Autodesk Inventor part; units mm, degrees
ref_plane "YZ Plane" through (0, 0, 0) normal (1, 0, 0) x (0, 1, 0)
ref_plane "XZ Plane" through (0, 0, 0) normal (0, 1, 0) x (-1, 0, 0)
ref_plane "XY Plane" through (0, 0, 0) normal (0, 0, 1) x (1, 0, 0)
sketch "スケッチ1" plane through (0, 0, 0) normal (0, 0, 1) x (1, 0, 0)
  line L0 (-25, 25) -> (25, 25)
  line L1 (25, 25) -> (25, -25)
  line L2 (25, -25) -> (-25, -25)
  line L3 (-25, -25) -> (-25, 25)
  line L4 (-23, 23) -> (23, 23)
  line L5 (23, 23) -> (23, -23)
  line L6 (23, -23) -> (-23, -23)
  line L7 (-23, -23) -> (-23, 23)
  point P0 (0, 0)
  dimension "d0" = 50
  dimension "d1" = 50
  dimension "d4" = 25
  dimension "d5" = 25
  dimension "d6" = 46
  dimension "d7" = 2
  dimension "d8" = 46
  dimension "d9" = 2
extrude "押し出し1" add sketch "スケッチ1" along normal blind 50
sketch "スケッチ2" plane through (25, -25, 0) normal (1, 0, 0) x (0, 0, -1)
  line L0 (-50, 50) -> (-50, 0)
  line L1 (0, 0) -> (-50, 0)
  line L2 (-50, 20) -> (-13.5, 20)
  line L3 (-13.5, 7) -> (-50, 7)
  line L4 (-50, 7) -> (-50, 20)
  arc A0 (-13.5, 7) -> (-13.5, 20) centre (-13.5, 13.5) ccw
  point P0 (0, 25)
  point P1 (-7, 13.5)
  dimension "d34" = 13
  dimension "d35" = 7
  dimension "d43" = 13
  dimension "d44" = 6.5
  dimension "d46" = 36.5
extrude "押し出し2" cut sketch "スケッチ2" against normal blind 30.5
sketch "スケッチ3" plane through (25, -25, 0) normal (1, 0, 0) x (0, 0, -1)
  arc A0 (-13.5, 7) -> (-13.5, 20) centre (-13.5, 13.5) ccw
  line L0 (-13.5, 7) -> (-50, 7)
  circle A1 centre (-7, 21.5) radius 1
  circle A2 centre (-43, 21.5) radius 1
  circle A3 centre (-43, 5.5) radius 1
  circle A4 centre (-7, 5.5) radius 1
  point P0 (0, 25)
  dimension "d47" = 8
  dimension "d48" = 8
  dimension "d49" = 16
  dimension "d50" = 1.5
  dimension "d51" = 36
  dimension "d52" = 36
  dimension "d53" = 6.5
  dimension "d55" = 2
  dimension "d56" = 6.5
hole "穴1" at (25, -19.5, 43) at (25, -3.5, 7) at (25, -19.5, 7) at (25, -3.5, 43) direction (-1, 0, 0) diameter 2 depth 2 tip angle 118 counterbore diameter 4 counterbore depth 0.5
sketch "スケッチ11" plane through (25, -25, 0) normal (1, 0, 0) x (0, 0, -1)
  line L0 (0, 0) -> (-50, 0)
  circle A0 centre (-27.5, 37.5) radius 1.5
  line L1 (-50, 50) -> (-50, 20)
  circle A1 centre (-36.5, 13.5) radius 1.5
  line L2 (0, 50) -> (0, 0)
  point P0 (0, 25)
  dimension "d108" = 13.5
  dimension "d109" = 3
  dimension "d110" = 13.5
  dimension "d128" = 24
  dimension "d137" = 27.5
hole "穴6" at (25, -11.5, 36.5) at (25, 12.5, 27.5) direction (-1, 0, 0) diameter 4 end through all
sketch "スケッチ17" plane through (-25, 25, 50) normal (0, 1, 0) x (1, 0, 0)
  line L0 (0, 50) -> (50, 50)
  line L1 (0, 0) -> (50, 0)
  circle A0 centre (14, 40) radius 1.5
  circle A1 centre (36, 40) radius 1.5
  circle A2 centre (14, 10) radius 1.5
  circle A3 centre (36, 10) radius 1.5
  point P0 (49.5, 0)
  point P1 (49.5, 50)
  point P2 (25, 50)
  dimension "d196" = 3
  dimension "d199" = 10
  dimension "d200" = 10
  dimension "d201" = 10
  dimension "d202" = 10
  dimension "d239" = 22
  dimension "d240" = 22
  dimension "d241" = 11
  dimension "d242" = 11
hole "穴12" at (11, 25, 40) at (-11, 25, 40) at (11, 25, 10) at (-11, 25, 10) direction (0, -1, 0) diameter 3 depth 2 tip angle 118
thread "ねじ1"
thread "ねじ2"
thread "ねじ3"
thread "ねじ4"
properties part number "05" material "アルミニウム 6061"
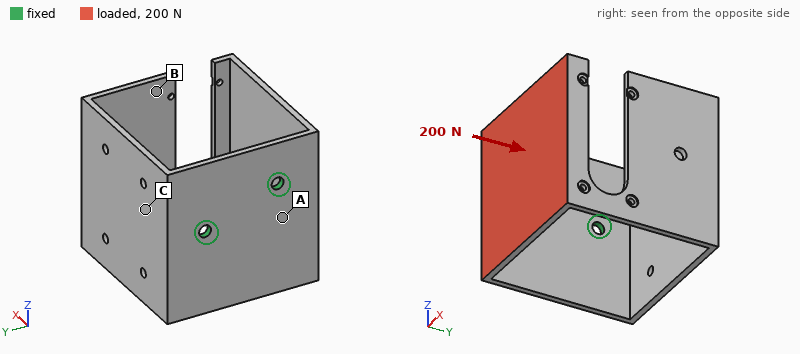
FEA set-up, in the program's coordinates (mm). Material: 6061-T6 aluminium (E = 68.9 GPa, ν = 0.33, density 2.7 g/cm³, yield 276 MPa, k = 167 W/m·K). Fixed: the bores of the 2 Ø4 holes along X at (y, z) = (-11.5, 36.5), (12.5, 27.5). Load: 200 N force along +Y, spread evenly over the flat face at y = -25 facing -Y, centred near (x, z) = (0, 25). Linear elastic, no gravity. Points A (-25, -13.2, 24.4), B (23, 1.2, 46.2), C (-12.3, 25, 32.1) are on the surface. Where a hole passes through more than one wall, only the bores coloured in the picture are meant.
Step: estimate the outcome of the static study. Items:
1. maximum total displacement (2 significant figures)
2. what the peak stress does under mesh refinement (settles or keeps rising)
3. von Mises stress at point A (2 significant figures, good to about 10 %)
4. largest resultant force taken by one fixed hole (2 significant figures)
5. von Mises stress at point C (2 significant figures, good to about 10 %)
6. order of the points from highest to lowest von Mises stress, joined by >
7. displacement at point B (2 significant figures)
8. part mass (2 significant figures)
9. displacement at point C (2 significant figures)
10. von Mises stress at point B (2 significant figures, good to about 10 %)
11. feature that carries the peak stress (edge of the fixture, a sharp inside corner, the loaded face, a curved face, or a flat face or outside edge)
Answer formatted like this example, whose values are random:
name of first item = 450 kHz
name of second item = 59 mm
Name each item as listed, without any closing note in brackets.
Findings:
maximum total displacement = 0.95 mm
what the peak stress does under mesh refinement = keeps rising
von Mises stress at point A = 48 MPa
largest resultant force taken by one fixed hole = 150 N
von Mises stress at point C = 26 MPa
order of the points from highest to lowest von Mises stress, joined by > = A > C > B
displacement at point B = 0.78 mm
part mass = 48 g
displacement at point C = 0.15 mm
von Mises stress at point B = 7.8 MPa
feature that carries the peak stress = edge of the fixture
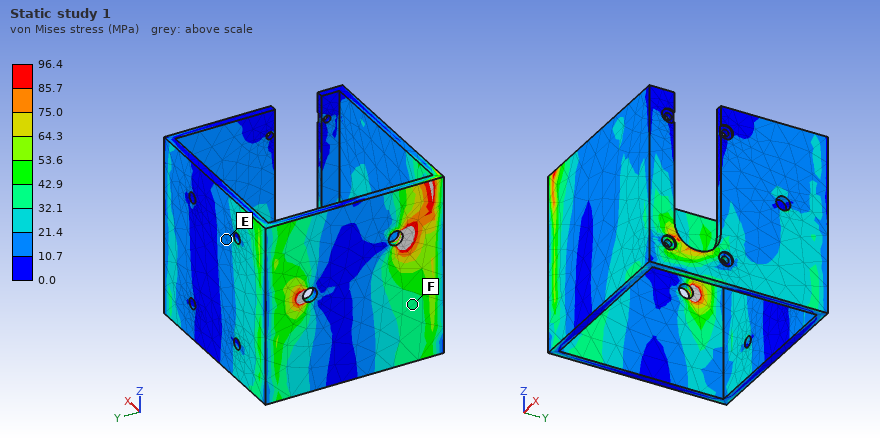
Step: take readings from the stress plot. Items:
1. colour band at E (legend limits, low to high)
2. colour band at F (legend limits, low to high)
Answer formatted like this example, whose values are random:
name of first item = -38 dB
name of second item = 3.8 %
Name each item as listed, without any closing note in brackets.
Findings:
colour band at E = 10.7 to 21.4 MPa
colour band at F = 32.1 to 42.9 MPa
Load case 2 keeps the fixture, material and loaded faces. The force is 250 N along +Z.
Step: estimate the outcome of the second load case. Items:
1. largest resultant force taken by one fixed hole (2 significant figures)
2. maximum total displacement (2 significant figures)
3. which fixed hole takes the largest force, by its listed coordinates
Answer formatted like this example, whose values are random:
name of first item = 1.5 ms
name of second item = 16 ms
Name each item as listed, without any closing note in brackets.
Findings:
largest resultant force taken by one fixed hole = 350 N
maximum total displacement = 0.89 mm
which fixed hole takes the largest force, by its listed coordinates = (-11.5, 36.5)
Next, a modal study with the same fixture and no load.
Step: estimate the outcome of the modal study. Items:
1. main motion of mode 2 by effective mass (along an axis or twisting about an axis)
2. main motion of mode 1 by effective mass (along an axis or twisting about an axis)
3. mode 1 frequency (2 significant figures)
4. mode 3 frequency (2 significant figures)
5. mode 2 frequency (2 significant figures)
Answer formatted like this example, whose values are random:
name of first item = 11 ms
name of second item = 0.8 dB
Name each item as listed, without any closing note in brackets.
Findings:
main motion of mode 2 by effective mass = along Z
main motion of mode 1 by effective mass = along Y
mode 1 frequency = 400 Hz
mode 3 frequency = 980 Hz
mode 2 frequency = 530 Hz
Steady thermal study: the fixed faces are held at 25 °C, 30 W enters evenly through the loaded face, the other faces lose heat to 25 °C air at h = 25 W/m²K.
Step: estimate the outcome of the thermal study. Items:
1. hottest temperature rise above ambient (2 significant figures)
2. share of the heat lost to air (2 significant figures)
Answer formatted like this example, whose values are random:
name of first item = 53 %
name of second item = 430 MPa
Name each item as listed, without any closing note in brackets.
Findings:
hottest temperature rise above ambient = 56 K
share of the heat lost to air = 25 %
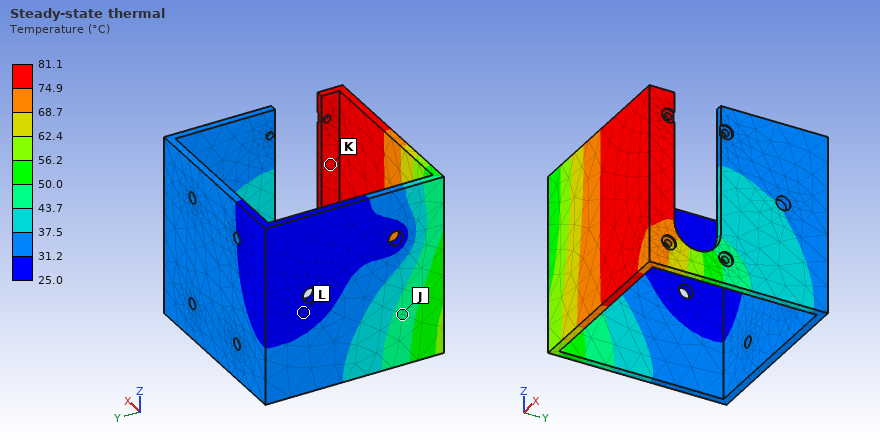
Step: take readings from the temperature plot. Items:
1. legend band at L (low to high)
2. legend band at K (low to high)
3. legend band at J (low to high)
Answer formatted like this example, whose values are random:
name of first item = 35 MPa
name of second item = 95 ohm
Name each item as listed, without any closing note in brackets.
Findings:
legend band at L = 25.0 to 31.2 °C
legend band at K = 74.9 to 81.1 °C
legend band at J = 43.7 to 50.0 °C
